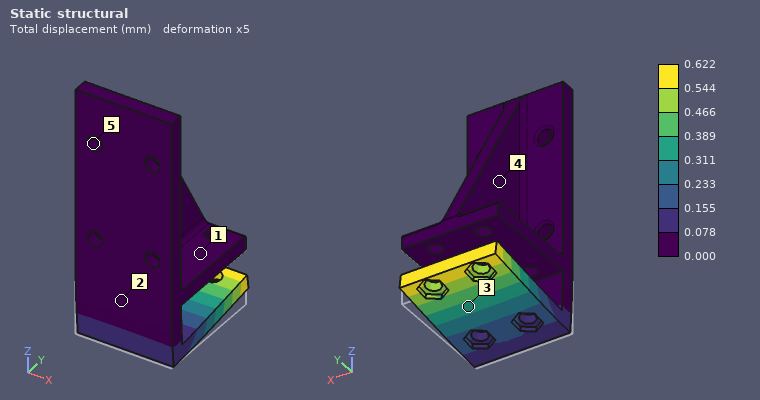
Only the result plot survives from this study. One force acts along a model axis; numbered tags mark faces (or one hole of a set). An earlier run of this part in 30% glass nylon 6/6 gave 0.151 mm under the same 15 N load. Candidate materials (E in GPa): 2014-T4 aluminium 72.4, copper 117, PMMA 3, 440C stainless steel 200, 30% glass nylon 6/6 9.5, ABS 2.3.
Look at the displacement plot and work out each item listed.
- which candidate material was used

ABS
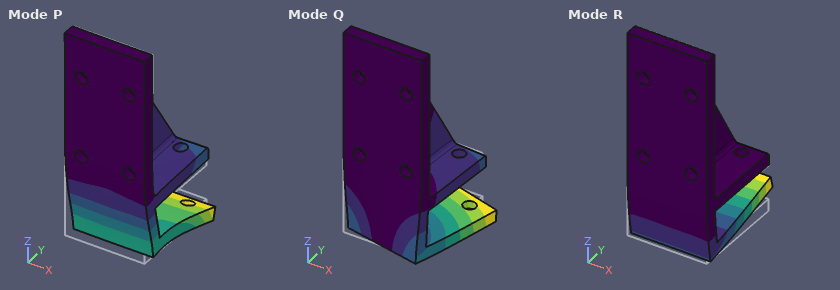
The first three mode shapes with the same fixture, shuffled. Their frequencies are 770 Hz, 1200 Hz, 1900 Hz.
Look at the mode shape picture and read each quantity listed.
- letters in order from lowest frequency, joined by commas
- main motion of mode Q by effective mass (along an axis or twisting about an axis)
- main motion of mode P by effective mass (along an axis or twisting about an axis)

R, Q, P
along X
along Y
